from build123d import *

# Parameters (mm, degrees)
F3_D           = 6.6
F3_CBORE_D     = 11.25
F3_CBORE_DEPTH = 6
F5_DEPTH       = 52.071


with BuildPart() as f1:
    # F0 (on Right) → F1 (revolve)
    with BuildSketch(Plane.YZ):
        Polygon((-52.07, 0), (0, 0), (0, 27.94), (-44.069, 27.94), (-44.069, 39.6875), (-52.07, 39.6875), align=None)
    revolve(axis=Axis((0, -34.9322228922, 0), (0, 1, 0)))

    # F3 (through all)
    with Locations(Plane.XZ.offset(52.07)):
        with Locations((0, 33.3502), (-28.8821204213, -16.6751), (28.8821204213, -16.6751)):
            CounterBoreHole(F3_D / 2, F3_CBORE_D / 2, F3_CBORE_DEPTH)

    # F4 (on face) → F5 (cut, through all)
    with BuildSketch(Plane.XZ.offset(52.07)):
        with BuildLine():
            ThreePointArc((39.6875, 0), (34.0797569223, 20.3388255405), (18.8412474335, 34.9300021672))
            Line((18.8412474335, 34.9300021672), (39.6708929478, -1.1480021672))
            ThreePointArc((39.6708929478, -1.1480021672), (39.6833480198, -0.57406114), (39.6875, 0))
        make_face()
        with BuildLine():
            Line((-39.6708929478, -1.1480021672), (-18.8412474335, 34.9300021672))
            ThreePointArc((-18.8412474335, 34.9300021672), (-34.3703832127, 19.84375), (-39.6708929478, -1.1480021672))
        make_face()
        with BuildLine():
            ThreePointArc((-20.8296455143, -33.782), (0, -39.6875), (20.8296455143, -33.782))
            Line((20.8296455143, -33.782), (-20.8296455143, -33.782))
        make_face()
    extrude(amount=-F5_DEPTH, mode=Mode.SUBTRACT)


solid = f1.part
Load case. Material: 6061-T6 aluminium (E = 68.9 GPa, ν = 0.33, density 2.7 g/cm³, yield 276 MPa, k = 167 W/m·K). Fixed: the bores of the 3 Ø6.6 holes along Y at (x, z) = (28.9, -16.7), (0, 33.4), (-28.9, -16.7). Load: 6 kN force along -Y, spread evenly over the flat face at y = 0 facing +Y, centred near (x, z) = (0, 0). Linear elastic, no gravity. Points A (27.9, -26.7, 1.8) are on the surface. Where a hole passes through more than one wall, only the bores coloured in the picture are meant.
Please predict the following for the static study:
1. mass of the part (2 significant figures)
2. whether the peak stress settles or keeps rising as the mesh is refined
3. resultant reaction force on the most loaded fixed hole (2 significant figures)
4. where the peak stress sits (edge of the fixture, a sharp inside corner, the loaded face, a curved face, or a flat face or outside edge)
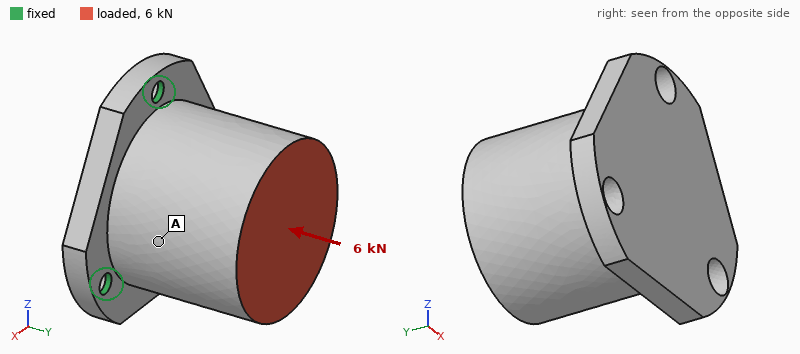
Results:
380 g
keeps rising
2.0 kN
edge of the fixture
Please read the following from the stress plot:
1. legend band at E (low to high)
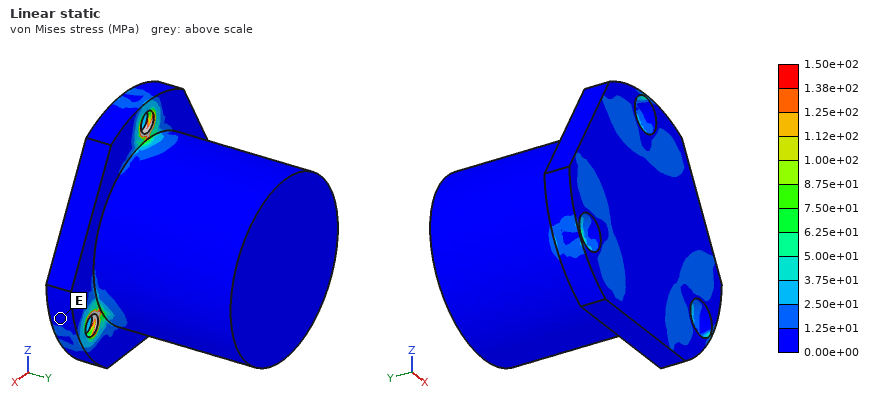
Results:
0.00e+00 to 1.25e+01 MPa
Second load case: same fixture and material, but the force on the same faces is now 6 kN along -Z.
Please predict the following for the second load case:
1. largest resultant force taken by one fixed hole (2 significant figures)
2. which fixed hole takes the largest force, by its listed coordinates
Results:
5.9 kN
(0, 33.4)
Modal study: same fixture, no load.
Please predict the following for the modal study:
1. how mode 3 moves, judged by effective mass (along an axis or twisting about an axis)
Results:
along Y
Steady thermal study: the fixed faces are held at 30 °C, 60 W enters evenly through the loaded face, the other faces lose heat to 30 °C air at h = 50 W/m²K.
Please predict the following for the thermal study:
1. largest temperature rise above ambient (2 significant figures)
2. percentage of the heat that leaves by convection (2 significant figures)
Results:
17 K
15 %
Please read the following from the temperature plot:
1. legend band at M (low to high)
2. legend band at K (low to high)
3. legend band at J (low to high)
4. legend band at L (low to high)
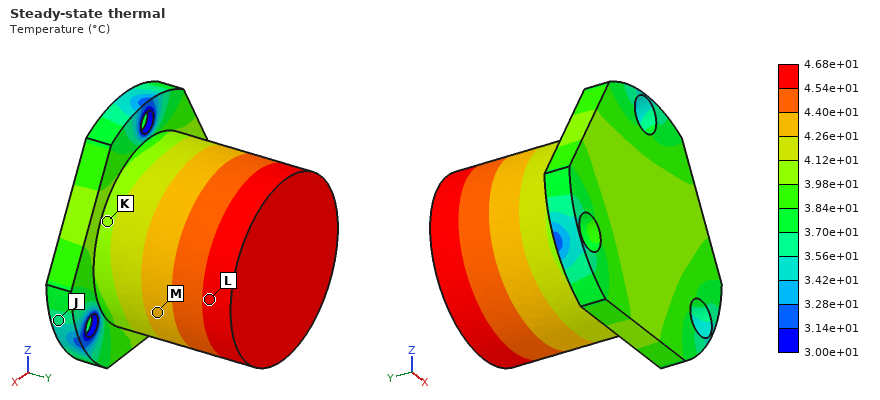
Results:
4.26e+01 to 4.40e+01 °C
3.98e+01 to 4.12e+01 °C
3.56e+01 to 3.70e+01 °C
4.54e+01 to 4.68e+01 °C
